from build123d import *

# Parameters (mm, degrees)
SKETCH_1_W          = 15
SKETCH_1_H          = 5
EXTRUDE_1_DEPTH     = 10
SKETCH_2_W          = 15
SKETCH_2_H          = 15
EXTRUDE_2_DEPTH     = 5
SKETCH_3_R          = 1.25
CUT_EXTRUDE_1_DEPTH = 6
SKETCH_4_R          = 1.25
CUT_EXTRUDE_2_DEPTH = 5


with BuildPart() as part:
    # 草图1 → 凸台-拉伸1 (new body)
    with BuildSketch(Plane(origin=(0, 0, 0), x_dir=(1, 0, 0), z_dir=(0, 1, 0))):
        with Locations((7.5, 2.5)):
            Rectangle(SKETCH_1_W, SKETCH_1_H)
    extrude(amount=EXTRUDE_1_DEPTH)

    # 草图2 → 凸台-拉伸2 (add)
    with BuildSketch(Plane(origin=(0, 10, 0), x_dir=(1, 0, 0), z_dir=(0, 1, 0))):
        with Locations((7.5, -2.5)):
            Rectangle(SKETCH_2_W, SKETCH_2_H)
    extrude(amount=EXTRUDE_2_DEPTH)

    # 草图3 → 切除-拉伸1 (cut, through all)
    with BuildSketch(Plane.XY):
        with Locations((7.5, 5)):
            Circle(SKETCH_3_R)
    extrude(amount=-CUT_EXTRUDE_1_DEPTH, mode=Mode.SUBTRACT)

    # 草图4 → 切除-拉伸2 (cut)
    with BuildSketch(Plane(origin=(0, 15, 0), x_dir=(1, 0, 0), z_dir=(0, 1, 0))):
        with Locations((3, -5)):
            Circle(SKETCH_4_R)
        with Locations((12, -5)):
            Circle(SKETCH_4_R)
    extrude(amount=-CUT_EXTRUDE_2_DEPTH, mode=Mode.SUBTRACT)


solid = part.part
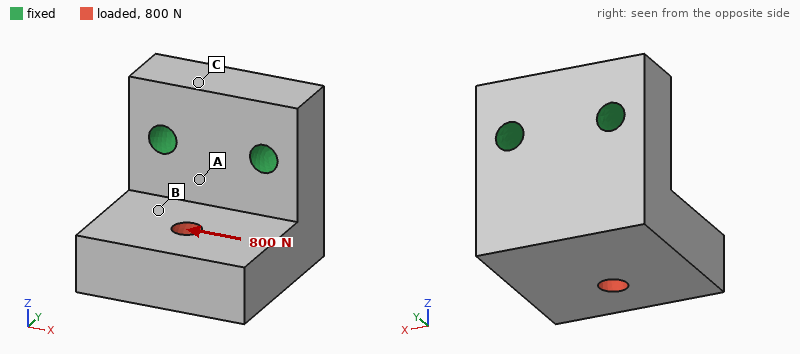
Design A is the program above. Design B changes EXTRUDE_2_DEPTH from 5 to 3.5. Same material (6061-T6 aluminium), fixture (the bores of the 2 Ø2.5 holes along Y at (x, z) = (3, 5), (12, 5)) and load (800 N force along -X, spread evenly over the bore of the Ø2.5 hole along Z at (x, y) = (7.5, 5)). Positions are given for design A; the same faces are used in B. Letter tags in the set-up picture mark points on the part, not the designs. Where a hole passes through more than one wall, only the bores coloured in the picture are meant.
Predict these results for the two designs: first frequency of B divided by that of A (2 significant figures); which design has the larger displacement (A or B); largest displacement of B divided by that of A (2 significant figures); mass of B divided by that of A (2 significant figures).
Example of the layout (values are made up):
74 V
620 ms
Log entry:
0.70
B
1.5
0.82
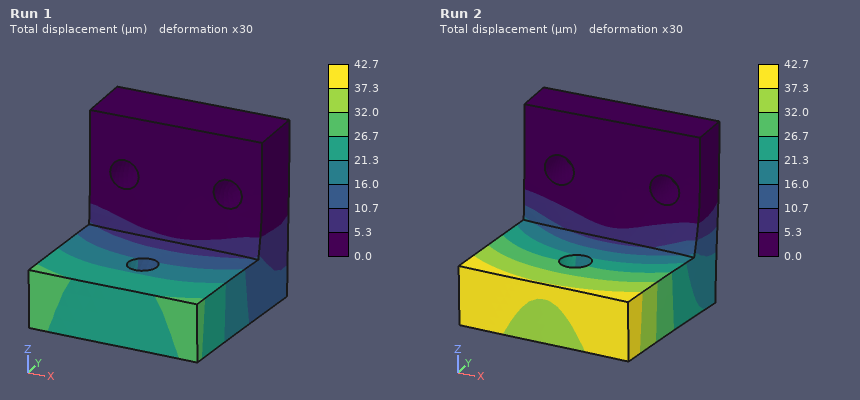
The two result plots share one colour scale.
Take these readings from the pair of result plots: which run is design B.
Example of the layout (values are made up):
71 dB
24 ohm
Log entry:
Run 2
